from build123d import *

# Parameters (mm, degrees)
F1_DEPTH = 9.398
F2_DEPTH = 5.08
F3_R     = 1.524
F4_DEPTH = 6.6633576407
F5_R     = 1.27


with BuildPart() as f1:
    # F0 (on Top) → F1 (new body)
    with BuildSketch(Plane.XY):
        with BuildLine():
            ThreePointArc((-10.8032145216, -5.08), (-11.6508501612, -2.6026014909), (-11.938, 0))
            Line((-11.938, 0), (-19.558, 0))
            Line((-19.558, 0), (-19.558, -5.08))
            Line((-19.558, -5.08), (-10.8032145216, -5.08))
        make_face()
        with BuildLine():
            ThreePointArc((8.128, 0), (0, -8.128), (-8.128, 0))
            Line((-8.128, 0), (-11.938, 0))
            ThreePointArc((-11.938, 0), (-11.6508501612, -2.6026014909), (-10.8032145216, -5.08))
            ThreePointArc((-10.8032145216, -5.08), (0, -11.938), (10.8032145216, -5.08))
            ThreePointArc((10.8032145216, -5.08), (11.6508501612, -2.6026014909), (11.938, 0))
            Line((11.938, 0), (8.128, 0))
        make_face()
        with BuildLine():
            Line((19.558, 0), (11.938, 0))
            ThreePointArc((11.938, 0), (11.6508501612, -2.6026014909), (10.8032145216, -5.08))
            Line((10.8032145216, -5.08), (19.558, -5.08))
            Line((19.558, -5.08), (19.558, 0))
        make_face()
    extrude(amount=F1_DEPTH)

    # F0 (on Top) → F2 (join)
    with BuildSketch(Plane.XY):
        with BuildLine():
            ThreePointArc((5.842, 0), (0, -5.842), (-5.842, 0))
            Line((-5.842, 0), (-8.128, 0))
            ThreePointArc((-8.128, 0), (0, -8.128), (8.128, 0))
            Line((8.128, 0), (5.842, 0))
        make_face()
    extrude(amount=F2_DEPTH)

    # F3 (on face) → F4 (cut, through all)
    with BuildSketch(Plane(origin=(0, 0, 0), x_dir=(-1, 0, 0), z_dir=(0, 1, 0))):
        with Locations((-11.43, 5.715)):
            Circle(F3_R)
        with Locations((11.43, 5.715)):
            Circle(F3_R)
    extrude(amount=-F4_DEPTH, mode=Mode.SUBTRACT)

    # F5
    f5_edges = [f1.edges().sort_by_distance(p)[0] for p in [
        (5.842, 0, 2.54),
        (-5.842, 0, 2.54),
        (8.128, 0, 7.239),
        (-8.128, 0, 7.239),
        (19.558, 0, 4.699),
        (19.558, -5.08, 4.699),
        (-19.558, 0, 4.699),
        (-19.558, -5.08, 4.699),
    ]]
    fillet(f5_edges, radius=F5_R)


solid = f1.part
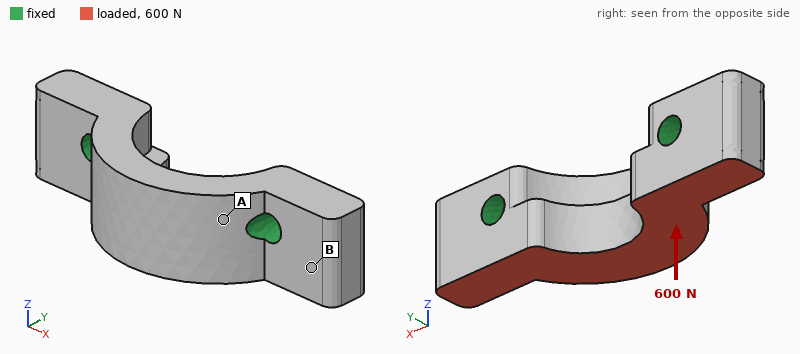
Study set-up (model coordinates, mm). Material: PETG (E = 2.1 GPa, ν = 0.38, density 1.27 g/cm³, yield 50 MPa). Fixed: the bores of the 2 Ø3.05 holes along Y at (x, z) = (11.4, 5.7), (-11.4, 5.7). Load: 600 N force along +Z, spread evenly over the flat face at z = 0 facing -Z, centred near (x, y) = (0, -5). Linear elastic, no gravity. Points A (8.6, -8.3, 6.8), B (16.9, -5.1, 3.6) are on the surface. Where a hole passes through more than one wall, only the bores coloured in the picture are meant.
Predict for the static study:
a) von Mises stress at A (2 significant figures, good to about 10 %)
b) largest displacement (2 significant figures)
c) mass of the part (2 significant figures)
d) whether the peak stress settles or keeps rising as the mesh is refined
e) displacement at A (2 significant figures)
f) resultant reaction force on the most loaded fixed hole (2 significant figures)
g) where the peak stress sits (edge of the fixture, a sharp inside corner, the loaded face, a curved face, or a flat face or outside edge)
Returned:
8.4 MPa
0.12 mm
2.6 g
keeps rising
0.045 mm
300 N
edge of the fixture
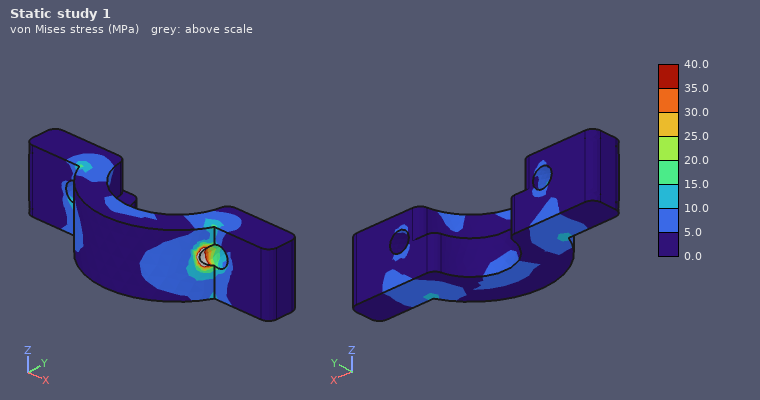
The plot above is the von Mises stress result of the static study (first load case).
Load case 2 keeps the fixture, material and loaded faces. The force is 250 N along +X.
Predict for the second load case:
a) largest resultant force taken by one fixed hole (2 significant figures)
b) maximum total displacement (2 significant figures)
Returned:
130 N
39 µm
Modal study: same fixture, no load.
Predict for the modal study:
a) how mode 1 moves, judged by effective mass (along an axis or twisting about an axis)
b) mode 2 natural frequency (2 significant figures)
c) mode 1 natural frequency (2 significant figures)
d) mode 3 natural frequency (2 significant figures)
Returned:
along Z
13 kHz
7900 Hz
13 kHz
